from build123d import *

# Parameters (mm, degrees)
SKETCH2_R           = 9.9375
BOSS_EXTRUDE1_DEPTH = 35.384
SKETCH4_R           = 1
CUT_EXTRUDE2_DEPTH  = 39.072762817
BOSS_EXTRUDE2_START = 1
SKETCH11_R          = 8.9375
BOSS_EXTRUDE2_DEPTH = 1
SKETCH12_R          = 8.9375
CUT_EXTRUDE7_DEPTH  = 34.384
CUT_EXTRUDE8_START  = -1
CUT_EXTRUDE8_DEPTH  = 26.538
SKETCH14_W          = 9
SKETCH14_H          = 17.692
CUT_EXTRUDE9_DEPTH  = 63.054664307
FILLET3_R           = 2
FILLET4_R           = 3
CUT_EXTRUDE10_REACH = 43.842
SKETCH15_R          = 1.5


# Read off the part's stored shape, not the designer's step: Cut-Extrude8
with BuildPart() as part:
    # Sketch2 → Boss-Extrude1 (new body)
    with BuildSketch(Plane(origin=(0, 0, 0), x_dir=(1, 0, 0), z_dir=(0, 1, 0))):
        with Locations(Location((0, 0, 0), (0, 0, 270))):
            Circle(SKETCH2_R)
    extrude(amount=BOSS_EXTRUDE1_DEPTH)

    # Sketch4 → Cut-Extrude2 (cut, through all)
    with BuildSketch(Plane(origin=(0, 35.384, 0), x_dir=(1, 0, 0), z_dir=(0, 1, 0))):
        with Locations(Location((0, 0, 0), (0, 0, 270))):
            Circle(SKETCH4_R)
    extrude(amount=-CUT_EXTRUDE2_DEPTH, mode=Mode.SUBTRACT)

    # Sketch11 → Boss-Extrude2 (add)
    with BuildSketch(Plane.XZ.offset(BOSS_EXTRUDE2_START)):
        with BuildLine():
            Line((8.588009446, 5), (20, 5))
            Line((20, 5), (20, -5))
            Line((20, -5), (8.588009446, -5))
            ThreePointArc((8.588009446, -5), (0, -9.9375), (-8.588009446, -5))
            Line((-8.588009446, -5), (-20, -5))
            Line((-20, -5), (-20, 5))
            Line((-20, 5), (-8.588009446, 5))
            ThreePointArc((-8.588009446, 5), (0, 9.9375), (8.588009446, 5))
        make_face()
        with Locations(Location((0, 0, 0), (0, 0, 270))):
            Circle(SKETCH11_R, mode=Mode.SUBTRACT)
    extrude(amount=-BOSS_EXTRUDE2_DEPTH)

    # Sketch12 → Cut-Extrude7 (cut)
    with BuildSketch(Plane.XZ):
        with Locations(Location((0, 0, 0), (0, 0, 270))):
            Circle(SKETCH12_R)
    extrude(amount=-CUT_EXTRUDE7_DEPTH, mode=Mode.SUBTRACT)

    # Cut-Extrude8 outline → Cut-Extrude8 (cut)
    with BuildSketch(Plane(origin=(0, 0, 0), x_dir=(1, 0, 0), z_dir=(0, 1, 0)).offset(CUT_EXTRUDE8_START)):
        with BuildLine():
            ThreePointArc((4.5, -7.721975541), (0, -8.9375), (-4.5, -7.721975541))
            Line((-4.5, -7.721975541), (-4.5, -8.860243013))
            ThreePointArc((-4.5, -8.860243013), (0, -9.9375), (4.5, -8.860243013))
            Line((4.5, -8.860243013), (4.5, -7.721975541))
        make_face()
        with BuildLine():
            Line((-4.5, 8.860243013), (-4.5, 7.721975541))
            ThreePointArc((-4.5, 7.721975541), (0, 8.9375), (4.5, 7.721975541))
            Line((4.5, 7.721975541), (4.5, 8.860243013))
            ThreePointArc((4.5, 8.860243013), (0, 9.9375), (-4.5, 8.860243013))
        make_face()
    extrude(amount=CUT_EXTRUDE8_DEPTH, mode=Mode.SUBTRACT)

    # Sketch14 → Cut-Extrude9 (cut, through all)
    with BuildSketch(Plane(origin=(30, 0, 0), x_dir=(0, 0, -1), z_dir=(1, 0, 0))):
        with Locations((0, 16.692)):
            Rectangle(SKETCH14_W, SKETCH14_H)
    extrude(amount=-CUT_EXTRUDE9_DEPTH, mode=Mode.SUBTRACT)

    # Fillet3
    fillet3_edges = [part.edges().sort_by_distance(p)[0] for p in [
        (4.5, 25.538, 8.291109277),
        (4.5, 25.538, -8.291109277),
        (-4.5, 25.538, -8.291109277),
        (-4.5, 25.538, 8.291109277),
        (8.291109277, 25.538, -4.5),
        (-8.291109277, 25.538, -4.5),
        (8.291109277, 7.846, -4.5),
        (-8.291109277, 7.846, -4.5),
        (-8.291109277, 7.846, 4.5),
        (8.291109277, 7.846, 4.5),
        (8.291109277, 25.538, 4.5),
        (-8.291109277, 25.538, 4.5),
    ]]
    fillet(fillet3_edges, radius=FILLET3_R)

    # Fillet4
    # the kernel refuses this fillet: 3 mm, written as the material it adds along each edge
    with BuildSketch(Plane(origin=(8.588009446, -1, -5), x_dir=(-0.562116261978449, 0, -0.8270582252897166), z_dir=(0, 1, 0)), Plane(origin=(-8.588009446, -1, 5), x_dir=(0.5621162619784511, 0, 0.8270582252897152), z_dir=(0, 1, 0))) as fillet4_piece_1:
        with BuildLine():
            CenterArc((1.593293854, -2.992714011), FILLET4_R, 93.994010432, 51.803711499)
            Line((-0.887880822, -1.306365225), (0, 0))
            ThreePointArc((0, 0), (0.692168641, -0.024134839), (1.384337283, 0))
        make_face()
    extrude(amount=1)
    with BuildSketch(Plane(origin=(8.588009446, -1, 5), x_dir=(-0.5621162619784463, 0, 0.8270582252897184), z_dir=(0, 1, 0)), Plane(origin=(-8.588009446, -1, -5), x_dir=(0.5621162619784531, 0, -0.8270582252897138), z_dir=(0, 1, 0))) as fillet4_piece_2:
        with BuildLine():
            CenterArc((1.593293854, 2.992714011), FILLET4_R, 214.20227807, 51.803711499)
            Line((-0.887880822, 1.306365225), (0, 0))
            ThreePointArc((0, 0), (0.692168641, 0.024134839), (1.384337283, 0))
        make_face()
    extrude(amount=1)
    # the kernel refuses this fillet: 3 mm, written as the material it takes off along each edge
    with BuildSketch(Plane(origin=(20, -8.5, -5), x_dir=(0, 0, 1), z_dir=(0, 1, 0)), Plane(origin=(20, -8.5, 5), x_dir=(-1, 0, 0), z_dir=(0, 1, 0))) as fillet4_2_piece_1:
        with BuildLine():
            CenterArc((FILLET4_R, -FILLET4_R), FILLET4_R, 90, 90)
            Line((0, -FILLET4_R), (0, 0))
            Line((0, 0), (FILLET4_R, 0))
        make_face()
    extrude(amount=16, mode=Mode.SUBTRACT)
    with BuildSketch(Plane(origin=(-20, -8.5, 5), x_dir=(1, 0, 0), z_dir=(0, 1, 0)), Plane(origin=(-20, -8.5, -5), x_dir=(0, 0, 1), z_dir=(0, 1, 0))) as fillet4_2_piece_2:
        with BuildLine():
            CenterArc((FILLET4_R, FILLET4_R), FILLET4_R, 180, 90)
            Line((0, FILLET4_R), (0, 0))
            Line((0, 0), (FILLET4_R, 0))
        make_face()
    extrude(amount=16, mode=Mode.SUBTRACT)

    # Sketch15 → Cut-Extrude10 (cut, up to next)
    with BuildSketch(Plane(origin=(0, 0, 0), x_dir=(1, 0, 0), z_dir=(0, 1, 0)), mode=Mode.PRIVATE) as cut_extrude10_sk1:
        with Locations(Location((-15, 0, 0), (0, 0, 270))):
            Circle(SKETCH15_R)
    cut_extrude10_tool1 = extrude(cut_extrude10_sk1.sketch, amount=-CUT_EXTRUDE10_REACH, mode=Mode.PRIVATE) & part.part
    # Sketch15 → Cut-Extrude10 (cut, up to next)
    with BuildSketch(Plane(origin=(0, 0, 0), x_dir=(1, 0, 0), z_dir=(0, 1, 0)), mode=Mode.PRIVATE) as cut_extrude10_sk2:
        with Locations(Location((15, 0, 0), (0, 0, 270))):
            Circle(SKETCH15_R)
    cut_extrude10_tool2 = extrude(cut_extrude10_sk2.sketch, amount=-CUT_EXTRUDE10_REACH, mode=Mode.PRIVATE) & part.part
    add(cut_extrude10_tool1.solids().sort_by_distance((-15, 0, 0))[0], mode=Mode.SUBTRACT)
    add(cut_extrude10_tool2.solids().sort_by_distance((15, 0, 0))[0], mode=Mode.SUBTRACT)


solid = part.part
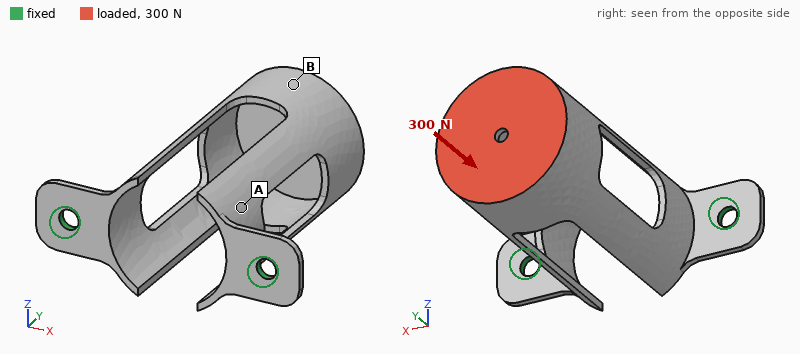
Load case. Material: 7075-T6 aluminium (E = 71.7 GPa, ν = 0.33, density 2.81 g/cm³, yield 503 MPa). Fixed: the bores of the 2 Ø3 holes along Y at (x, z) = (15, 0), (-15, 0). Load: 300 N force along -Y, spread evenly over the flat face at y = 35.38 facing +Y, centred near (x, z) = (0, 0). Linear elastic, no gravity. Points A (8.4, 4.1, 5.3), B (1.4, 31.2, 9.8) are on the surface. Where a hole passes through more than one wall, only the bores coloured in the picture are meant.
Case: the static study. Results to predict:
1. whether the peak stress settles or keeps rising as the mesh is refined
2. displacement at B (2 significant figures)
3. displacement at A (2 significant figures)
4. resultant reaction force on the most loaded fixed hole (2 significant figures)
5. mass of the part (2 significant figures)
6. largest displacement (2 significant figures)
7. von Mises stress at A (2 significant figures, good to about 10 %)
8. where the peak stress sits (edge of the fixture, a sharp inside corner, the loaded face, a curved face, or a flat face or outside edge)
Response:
keeps rising
56 µm
55 µm
150 N
5.0 g
88 µm
35 MPa
edge of the fixture
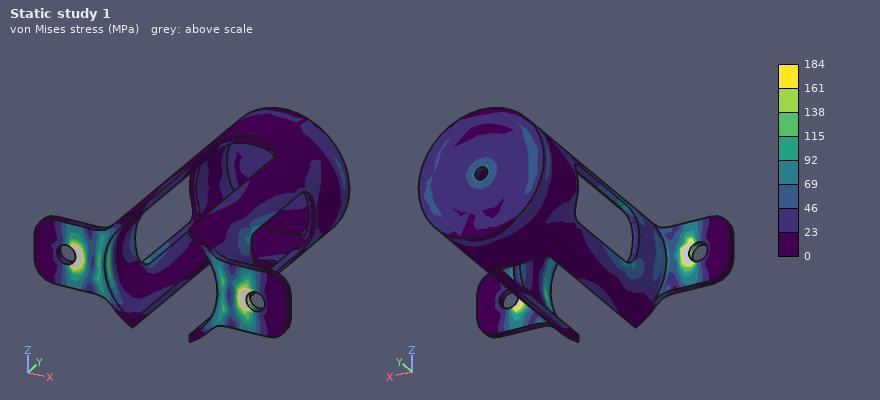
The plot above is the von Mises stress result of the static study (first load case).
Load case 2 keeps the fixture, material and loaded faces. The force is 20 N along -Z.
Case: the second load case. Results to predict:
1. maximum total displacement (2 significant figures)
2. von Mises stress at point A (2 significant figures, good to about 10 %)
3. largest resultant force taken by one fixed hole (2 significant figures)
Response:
0.56 mm
18 MPa
10 N
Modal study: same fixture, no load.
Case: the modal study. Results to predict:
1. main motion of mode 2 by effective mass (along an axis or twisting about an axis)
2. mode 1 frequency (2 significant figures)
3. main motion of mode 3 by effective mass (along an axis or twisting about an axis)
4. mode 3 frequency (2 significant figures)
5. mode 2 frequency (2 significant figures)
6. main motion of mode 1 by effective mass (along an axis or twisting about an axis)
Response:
along X
630 Hz
twisting about Y
3600 Hz
2100 Hz
along Z
